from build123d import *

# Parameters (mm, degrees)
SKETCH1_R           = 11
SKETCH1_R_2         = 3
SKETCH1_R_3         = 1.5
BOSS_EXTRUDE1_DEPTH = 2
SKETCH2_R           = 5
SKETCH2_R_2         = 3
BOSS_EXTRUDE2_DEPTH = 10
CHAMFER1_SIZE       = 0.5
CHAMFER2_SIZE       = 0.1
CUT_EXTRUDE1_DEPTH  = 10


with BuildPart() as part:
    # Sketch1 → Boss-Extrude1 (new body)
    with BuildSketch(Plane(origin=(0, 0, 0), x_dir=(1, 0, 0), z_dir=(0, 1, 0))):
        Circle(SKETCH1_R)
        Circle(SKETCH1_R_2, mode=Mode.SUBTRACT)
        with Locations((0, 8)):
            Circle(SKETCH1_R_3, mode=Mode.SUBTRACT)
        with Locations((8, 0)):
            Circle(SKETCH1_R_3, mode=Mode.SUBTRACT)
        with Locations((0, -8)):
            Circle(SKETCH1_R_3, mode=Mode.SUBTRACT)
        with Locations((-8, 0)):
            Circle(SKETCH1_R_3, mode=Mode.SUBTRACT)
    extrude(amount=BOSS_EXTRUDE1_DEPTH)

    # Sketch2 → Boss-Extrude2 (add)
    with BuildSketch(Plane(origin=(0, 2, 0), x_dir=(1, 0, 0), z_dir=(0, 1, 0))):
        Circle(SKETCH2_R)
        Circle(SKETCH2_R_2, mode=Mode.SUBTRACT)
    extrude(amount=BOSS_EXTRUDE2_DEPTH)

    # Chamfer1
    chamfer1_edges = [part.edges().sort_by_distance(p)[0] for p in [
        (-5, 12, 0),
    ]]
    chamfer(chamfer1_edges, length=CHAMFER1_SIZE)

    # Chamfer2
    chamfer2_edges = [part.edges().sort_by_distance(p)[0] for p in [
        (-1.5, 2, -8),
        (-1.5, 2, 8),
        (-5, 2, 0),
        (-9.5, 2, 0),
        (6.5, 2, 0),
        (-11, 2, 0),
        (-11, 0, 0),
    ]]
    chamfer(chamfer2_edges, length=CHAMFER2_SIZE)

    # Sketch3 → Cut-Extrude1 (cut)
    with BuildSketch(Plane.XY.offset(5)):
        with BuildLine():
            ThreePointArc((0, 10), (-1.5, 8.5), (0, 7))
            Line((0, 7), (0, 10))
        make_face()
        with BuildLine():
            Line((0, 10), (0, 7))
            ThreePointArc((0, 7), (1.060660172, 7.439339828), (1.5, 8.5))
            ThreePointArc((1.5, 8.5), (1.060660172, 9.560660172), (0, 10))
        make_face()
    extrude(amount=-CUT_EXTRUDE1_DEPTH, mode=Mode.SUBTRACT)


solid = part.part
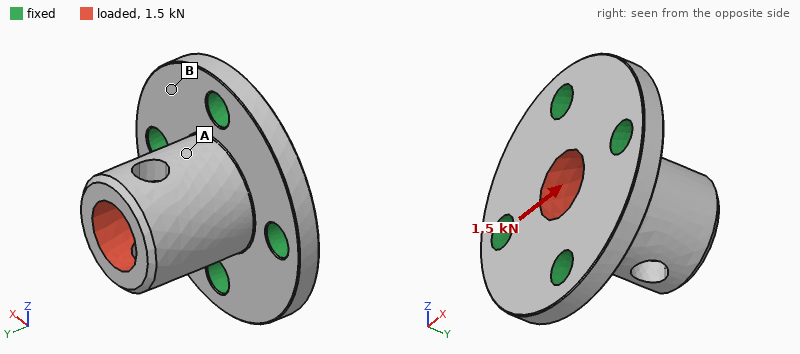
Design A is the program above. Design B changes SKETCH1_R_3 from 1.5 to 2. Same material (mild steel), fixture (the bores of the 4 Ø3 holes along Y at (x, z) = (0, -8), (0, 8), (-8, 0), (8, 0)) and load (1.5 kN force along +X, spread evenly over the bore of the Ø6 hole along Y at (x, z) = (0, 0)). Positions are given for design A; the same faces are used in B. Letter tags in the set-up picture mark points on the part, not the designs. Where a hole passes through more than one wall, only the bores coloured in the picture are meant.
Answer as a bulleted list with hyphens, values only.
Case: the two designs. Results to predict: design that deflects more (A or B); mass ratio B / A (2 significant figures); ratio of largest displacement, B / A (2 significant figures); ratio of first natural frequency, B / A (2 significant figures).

- A
- 0.96
- 0.86
- 1.1
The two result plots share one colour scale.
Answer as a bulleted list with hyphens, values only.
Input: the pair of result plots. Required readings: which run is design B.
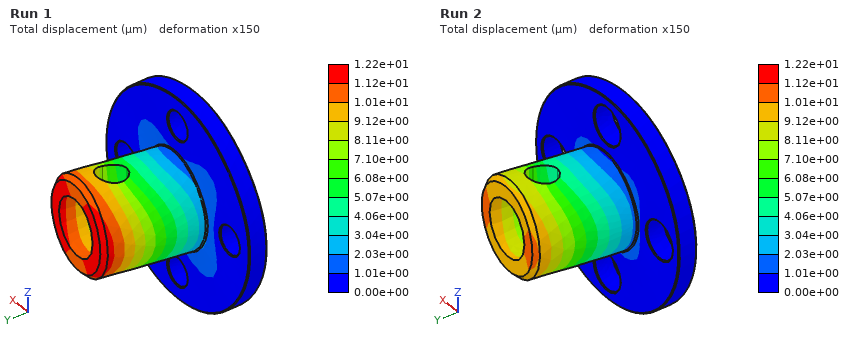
- Run 2
